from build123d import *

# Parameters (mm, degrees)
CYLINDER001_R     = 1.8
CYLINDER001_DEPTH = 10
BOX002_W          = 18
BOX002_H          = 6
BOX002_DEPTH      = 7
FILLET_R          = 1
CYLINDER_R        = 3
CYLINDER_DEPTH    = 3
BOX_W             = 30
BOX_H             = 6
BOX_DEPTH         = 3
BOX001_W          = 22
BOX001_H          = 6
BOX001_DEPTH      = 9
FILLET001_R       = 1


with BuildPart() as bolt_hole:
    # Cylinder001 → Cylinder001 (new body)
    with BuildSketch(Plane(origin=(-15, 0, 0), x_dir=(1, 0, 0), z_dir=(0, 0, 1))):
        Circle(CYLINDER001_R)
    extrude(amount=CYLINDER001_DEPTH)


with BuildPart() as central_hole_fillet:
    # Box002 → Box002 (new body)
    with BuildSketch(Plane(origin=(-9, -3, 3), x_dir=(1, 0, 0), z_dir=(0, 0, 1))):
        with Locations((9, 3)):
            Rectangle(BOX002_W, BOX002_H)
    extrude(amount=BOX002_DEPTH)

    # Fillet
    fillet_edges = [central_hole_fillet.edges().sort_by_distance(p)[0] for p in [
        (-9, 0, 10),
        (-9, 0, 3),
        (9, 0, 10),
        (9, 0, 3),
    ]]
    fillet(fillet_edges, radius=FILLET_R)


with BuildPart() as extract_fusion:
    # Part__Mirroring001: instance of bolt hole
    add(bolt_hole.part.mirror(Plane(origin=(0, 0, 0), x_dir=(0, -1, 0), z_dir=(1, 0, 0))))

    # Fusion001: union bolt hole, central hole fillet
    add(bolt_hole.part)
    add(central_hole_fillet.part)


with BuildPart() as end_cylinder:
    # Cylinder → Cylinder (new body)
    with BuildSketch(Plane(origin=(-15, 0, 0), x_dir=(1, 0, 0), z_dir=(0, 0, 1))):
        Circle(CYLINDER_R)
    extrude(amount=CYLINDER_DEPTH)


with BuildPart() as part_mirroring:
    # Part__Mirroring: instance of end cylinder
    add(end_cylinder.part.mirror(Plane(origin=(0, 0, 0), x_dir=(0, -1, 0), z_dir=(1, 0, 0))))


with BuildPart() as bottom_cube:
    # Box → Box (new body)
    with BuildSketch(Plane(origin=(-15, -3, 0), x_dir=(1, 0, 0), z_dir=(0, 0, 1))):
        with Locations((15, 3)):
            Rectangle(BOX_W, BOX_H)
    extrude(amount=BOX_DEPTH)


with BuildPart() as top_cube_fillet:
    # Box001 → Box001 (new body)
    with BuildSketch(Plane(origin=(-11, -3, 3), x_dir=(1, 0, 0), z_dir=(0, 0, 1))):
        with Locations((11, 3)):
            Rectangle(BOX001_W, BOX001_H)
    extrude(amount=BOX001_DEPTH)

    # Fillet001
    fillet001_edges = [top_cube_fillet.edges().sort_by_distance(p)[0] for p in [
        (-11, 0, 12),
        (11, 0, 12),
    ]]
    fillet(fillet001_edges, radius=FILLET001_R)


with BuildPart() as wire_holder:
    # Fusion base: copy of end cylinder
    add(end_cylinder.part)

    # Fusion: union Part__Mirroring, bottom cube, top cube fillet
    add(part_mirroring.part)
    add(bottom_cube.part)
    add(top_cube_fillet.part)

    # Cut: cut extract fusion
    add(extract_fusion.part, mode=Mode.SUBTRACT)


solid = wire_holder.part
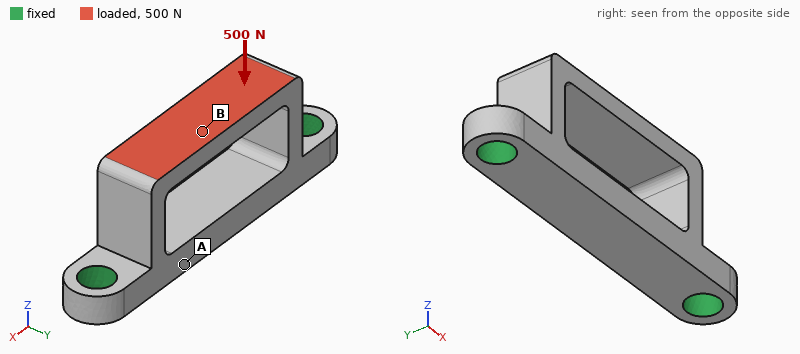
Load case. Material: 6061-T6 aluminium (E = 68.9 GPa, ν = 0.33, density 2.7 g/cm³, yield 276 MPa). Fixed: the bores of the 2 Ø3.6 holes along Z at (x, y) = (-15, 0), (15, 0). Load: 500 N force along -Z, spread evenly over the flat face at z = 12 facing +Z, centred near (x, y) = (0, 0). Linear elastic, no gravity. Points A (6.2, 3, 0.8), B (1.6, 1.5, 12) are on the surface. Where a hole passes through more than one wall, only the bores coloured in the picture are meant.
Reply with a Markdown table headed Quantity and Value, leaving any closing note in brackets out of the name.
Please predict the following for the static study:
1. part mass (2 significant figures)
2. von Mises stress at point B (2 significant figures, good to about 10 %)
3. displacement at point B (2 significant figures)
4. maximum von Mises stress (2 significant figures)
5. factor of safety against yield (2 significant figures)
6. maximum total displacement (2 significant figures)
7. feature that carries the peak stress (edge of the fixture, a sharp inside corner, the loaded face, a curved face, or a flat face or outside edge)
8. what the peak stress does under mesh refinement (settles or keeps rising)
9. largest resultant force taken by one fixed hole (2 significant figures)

| Quantity | Value |
|---|---|
| part mass | 2.7 g |
| von Mises stress at point B | 120 MPa |
| displacement at point B | 54 µm |
| maximum von Mises stress | 220 MPa |
| factor of safety against yield | 1.3 |
| maximum total displacement | 58 µm |
| feature that carries the peak stress | a curved face |
| what the peak stress does under mesh refinement | settles |
| largest resultant force taken by one fixed hole | 270 N |
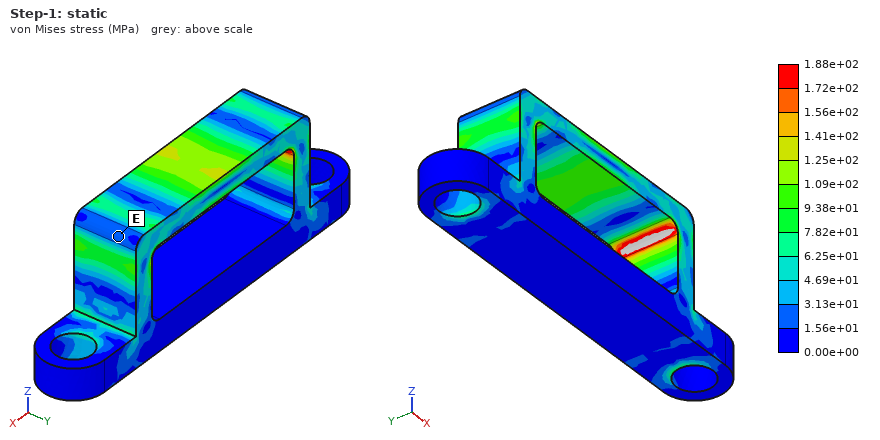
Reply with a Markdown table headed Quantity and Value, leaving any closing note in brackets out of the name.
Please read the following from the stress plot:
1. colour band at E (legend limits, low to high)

| Quantity | Value |
|---|---|
| colour band at E | 1.56e+01 to 3.13e+01 MPa |
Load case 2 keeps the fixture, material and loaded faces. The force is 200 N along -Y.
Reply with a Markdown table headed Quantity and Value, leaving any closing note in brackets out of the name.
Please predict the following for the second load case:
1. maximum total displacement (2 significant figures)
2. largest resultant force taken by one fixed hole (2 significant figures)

| Quantity | Value |
|---|---|
| maximum total displacement | 58 µm |
| largest resultant force taken by one fixed hole | 100 N |
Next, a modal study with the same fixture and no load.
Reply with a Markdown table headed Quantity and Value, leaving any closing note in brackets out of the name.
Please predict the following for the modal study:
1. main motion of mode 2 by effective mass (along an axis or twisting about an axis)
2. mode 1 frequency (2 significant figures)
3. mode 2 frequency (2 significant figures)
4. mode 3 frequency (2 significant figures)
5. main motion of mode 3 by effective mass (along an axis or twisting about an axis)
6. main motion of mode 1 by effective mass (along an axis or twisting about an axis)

| Quantity | Value |
|---|---|
| main motion of mode 2 by effective mass | along X |
| mode 1 frequency | 12 kHz |
| mode 2 frequency | 13 kHz |
| mode 3 frequency | 21 kHz |
| main motion of mode 3 by effective mass | along Z |
| main motion of mode 1 by effective mass | along Y |
